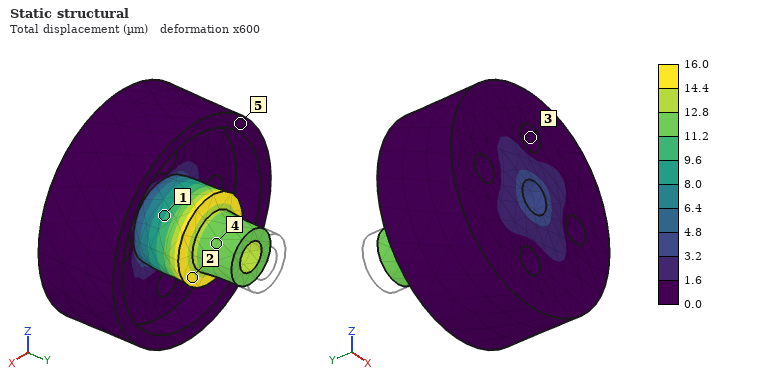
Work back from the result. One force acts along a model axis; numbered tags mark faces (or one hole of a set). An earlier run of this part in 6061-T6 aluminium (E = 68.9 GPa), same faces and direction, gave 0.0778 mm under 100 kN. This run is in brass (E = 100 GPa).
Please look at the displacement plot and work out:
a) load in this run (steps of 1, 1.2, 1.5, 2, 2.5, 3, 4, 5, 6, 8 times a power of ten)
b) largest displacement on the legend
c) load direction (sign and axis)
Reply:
30 kN
16.0 µm
-Y
